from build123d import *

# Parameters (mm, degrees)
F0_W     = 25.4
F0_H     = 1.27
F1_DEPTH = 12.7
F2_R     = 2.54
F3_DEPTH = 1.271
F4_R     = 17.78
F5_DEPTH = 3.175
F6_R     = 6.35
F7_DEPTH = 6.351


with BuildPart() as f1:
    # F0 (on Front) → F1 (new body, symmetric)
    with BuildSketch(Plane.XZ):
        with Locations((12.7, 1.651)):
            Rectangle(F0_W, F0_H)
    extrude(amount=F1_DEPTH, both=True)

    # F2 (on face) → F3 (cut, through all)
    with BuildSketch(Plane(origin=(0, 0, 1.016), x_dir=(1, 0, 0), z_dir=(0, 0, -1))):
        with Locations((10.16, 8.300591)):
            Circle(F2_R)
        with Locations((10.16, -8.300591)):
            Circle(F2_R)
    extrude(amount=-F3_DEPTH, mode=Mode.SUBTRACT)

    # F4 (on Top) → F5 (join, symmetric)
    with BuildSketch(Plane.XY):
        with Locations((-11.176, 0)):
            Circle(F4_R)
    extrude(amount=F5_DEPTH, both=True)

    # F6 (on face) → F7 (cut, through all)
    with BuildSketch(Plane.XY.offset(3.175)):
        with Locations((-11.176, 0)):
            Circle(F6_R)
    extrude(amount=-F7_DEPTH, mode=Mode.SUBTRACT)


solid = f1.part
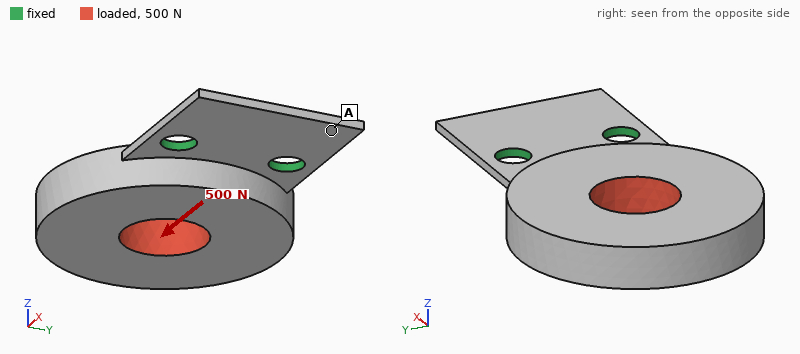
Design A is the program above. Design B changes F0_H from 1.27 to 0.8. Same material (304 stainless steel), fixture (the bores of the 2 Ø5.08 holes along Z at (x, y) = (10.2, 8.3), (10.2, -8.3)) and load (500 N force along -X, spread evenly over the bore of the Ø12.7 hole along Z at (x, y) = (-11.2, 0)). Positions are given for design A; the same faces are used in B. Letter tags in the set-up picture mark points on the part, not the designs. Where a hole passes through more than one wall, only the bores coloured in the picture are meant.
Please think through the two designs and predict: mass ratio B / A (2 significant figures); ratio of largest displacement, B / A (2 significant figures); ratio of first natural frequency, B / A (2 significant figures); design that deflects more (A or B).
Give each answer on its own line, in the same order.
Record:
0.96
3.5
0.54
B
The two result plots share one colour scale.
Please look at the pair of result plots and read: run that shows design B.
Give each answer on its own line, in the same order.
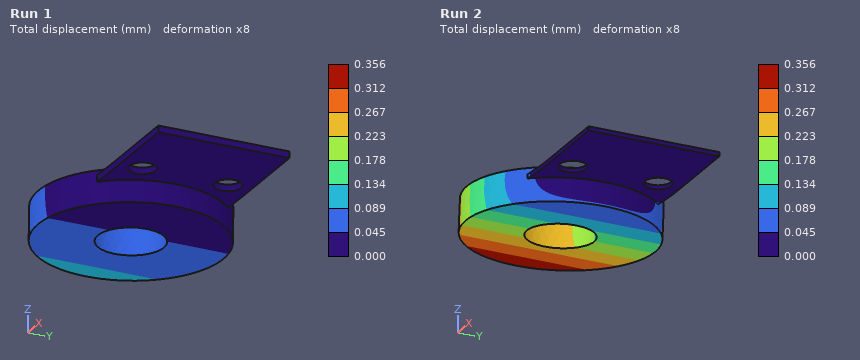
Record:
Run 2
